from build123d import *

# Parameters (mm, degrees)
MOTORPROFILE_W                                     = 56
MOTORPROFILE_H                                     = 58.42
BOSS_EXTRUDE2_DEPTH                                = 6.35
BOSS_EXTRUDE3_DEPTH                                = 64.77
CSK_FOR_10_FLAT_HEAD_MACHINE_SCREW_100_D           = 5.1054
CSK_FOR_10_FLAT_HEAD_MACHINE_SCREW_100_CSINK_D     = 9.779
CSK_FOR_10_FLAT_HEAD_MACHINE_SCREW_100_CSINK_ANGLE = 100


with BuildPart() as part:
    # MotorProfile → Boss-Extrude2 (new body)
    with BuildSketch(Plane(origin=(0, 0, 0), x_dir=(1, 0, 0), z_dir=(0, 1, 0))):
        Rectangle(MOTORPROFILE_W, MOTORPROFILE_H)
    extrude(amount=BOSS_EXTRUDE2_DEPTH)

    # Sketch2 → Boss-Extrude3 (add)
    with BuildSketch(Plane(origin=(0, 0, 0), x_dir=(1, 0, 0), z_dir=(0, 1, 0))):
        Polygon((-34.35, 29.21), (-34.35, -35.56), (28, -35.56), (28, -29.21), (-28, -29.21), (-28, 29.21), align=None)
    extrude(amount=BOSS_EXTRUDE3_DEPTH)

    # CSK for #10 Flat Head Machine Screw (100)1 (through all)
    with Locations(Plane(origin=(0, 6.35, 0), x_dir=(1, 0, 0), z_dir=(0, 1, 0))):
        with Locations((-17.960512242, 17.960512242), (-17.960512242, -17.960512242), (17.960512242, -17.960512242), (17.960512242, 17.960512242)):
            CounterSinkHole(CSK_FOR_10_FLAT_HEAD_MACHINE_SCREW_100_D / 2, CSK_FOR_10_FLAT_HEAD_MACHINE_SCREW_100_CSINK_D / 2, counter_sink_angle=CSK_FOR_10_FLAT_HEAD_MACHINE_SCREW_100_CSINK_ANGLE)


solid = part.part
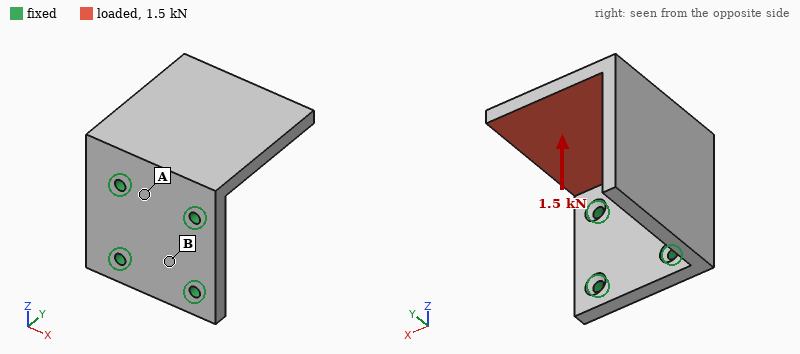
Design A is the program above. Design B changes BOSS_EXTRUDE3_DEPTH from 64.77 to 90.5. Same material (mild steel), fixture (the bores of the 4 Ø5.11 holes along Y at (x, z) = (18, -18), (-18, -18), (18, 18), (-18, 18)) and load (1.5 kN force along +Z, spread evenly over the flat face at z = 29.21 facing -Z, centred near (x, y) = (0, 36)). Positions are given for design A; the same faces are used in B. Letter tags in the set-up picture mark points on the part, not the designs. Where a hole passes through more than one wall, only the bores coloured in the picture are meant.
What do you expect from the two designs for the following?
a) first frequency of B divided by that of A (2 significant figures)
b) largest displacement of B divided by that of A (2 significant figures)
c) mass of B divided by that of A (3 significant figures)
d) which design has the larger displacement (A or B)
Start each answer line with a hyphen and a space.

- 0.65
- 1.6
- 1.28
- B
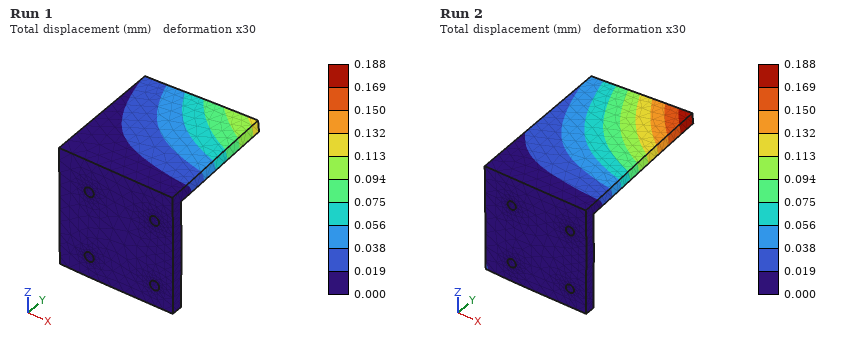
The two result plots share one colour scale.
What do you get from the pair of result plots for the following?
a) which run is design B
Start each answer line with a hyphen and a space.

- Run 2
